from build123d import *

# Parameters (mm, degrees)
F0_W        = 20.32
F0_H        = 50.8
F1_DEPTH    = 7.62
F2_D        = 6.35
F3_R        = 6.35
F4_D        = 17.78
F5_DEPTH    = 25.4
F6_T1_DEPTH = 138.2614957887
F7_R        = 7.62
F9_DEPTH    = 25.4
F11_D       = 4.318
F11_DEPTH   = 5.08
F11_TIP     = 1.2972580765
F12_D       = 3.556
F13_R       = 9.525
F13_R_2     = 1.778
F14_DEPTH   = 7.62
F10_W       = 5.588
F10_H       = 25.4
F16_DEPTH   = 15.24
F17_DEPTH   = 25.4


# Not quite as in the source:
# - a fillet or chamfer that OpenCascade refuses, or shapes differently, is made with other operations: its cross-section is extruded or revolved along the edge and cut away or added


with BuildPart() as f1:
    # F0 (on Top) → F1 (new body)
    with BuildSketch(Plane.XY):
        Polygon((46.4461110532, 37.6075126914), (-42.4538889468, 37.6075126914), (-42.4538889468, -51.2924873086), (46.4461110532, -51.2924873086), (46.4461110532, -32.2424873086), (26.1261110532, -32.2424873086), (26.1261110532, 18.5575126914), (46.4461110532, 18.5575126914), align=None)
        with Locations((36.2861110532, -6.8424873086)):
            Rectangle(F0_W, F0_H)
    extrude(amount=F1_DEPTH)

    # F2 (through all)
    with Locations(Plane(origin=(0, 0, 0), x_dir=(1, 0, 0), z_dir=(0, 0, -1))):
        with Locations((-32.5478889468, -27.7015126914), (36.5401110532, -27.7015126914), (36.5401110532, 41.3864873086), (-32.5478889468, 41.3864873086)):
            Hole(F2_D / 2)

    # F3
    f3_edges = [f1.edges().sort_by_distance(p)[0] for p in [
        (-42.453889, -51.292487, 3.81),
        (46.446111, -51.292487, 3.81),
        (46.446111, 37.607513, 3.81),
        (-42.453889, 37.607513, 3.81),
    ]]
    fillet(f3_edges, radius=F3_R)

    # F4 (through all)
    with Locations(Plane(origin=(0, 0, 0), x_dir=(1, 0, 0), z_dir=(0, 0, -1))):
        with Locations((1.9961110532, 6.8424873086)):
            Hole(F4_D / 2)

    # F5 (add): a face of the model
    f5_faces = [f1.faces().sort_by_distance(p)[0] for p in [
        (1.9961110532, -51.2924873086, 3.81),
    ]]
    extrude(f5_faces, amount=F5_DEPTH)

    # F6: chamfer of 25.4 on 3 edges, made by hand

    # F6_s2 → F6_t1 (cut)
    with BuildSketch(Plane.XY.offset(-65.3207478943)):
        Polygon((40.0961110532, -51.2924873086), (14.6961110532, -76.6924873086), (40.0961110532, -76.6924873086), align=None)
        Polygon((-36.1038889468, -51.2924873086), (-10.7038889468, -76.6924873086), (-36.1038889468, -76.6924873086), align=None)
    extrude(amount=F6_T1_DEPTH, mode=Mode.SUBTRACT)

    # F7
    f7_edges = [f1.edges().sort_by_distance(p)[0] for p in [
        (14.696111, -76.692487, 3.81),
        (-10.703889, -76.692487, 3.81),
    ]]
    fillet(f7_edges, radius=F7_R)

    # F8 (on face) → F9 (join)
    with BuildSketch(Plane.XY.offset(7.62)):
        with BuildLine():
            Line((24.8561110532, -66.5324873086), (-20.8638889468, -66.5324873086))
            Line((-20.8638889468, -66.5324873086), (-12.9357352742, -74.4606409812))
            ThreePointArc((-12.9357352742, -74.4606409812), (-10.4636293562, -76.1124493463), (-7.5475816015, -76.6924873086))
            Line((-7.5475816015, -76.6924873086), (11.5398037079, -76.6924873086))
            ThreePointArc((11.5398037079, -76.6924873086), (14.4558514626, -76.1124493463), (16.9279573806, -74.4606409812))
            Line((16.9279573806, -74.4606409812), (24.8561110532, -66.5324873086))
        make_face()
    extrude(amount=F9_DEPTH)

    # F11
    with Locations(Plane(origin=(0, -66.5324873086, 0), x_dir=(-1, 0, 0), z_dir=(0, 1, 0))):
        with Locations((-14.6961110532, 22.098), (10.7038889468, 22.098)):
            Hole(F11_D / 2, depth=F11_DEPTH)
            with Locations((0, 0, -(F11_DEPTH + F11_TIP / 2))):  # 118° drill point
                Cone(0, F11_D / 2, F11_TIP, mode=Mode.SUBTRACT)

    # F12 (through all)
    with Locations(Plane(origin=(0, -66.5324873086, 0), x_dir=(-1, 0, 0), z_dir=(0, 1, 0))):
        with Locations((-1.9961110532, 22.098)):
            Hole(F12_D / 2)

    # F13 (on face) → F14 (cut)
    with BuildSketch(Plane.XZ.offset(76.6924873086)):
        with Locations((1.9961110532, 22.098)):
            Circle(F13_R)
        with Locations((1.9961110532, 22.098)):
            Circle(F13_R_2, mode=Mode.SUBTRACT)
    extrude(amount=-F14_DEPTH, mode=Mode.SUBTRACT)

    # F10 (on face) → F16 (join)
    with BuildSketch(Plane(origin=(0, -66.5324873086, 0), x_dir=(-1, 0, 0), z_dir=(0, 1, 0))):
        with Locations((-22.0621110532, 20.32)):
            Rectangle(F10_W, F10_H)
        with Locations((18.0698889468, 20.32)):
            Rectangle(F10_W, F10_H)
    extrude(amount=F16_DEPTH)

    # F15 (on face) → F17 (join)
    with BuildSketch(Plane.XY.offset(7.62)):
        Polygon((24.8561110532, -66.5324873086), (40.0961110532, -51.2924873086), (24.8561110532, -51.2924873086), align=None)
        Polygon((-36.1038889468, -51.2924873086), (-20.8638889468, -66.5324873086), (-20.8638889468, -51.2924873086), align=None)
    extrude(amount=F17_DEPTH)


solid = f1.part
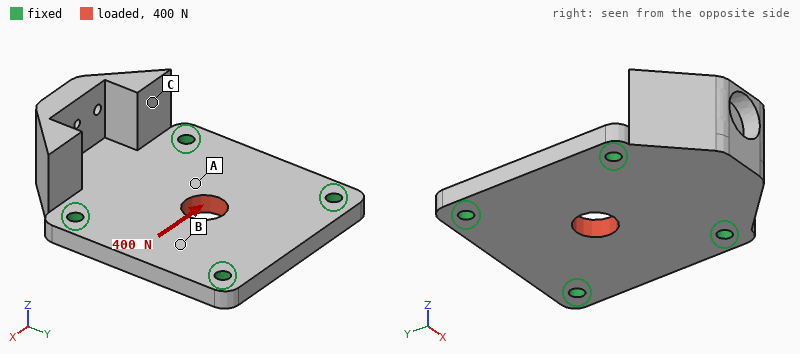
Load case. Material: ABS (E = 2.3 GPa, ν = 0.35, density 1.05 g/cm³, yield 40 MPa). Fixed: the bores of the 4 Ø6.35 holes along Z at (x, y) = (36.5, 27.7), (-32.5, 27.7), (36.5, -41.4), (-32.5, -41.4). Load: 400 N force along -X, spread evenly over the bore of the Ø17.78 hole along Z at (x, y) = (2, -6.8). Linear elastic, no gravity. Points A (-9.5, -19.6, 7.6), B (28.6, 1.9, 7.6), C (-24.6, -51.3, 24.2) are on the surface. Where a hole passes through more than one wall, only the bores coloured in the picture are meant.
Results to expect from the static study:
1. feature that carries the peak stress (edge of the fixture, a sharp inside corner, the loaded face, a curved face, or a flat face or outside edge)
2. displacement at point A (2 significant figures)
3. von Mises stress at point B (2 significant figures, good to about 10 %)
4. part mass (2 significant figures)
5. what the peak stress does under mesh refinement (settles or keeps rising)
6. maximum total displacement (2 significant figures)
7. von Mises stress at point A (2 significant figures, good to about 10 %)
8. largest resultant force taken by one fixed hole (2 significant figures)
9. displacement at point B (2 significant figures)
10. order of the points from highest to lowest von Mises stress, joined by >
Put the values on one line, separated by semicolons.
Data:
edge of the fixture; 12 µm; 0.42 MPa; 88 g; keeps rising; 17 µm; 0.71 MPa; 110 N; 11 µm; A > B > C
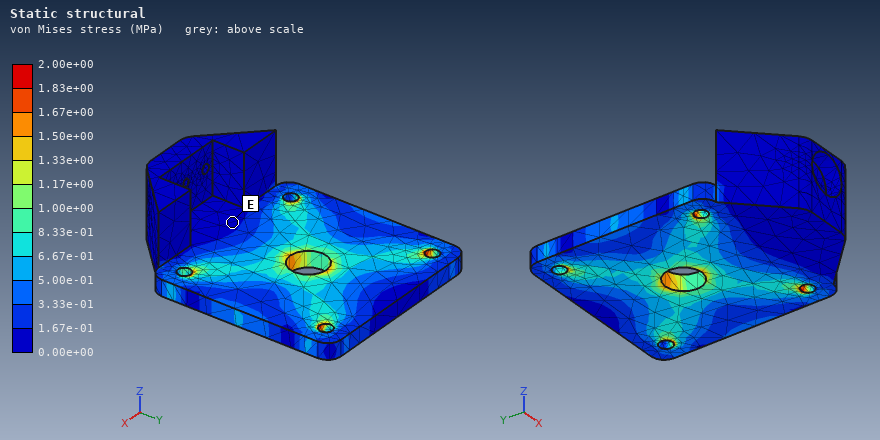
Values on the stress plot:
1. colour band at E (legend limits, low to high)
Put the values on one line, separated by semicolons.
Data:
0.00e+00 to 1.67e-01 MPa
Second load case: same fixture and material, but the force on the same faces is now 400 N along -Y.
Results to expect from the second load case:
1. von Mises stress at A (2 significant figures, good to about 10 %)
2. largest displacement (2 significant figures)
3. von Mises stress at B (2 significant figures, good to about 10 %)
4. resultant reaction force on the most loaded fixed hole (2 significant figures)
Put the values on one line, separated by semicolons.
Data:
0.71 MPa; 17 µm; 0.37 MPa; 110 N
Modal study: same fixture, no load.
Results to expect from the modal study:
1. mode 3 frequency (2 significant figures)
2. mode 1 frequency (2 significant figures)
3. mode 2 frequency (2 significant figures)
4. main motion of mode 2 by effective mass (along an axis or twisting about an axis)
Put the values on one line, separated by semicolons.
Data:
1900 Hz; 750 Hz; 1700 Hz; along Z
